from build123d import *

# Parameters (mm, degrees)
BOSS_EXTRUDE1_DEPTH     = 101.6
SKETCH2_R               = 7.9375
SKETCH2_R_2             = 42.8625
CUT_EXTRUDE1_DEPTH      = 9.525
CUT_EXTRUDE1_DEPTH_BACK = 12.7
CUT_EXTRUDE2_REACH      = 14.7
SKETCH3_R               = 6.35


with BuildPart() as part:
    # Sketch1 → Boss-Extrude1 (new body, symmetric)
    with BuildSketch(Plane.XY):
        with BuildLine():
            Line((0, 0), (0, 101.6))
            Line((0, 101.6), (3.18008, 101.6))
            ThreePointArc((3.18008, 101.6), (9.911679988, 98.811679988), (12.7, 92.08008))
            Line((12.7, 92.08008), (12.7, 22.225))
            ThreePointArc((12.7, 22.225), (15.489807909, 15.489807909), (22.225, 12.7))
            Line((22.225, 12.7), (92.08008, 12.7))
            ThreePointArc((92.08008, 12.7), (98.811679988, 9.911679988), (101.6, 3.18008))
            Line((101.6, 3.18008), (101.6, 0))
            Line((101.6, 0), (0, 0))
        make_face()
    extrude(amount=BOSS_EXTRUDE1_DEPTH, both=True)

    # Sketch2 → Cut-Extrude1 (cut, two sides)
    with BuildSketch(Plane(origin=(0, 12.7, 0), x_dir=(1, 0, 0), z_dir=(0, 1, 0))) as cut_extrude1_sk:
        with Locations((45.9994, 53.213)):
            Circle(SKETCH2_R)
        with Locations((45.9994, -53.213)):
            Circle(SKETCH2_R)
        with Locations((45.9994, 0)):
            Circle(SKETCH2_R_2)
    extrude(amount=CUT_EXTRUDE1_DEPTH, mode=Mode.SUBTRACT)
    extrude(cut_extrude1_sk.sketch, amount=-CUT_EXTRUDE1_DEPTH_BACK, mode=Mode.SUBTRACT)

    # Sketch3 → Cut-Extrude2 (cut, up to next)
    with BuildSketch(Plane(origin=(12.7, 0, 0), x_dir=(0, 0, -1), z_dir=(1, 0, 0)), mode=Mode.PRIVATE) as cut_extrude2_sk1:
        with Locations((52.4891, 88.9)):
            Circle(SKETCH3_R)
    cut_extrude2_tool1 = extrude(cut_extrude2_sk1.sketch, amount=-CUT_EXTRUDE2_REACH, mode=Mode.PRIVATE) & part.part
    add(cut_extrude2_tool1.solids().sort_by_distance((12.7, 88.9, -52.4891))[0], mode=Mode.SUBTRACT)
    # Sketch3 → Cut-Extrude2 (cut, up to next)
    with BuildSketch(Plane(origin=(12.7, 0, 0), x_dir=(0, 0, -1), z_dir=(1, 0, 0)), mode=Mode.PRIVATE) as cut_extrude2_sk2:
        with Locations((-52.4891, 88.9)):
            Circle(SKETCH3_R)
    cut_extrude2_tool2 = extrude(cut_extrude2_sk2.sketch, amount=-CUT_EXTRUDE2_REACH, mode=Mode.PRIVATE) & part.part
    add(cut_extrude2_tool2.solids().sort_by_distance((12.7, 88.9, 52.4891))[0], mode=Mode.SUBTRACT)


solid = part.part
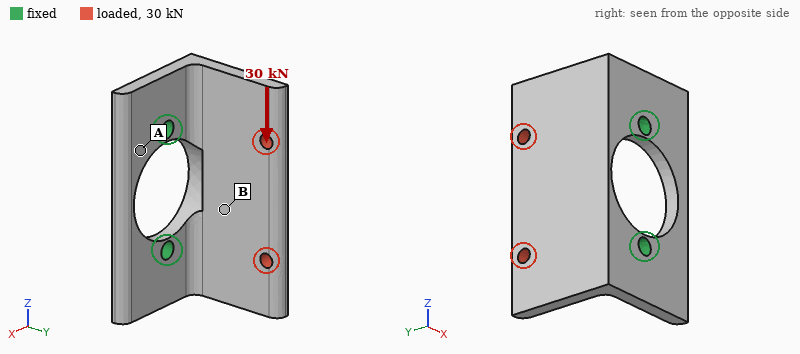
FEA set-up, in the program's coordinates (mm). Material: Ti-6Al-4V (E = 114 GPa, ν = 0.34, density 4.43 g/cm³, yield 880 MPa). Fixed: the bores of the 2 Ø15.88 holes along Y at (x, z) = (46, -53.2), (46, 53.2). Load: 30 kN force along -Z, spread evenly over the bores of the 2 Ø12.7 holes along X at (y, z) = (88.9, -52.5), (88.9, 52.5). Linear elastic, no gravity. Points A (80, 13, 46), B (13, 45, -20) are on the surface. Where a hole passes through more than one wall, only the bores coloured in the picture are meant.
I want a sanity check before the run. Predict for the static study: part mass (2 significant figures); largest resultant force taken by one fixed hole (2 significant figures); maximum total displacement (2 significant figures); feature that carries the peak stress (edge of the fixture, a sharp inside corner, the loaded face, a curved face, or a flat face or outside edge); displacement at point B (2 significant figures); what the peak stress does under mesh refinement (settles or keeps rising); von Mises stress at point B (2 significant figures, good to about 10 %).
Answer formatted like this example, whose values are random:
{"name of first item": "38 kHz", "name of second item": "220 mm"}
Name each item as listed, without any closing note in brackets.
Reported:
{"part mass": "1.8 kg", "largest resultant force taken by one fixed hole": "25 kN", "maximum total displacement": "0.68 mm", "feature that carries the peak stress": "edge of the fixture", "displacement at point B": "0.23 mm", "what the peak stress does under mesh refinement": "keeps rising", "von Mises stress at point B": "87 MPa"}
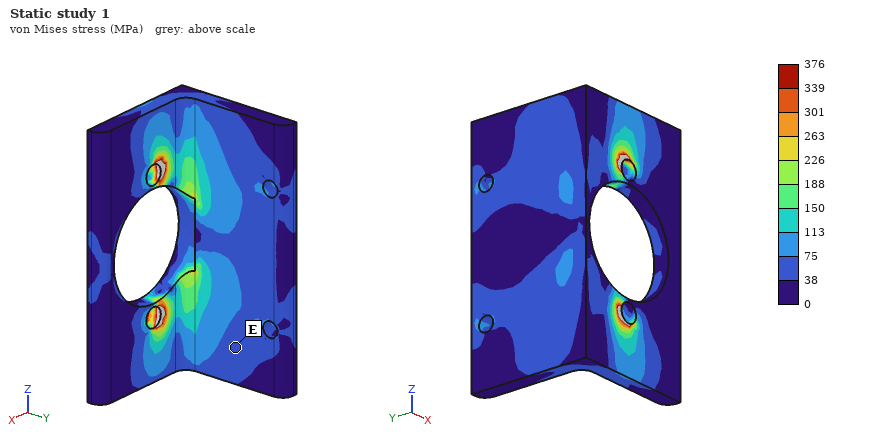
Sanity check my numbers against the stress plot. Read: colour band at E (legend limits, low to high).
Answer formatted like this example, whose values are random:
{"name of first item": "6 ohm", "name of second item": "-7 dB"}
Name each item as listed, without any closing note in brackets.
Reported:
{"colour band at E": "38 to 75 MPa"}
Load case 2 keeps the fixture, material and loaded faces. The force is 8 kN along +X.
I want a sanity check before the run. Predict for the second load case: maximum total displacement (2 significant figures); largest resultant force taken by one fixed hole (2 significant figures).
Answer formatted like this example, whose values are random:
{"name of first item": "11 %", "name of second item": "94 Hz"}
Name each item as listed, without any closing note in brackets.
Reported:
{"maximum total displacement": "1.3 mm", "largest resultant force taken by one fixed hole": "4.0 kN"}
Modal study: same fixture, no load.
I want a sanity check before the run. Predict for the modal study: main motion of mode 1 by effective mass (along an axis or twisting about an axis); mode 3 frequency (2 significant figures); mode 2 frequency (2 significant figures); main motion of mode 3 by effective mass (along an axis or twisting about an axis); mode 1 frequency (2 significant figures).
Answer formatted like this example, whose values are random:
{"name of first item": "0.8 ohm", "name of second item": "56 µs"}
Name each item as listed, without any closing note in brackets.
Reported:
{"main motion of mode 1 by effective mass": "along X", "mode 3 frequency": "2000 Hz", "mode 2 frequency": "1200 Hz", "main motion of mode 3 by effective mass": "along Z", "mode 1 frequency": "640 Hz"}
